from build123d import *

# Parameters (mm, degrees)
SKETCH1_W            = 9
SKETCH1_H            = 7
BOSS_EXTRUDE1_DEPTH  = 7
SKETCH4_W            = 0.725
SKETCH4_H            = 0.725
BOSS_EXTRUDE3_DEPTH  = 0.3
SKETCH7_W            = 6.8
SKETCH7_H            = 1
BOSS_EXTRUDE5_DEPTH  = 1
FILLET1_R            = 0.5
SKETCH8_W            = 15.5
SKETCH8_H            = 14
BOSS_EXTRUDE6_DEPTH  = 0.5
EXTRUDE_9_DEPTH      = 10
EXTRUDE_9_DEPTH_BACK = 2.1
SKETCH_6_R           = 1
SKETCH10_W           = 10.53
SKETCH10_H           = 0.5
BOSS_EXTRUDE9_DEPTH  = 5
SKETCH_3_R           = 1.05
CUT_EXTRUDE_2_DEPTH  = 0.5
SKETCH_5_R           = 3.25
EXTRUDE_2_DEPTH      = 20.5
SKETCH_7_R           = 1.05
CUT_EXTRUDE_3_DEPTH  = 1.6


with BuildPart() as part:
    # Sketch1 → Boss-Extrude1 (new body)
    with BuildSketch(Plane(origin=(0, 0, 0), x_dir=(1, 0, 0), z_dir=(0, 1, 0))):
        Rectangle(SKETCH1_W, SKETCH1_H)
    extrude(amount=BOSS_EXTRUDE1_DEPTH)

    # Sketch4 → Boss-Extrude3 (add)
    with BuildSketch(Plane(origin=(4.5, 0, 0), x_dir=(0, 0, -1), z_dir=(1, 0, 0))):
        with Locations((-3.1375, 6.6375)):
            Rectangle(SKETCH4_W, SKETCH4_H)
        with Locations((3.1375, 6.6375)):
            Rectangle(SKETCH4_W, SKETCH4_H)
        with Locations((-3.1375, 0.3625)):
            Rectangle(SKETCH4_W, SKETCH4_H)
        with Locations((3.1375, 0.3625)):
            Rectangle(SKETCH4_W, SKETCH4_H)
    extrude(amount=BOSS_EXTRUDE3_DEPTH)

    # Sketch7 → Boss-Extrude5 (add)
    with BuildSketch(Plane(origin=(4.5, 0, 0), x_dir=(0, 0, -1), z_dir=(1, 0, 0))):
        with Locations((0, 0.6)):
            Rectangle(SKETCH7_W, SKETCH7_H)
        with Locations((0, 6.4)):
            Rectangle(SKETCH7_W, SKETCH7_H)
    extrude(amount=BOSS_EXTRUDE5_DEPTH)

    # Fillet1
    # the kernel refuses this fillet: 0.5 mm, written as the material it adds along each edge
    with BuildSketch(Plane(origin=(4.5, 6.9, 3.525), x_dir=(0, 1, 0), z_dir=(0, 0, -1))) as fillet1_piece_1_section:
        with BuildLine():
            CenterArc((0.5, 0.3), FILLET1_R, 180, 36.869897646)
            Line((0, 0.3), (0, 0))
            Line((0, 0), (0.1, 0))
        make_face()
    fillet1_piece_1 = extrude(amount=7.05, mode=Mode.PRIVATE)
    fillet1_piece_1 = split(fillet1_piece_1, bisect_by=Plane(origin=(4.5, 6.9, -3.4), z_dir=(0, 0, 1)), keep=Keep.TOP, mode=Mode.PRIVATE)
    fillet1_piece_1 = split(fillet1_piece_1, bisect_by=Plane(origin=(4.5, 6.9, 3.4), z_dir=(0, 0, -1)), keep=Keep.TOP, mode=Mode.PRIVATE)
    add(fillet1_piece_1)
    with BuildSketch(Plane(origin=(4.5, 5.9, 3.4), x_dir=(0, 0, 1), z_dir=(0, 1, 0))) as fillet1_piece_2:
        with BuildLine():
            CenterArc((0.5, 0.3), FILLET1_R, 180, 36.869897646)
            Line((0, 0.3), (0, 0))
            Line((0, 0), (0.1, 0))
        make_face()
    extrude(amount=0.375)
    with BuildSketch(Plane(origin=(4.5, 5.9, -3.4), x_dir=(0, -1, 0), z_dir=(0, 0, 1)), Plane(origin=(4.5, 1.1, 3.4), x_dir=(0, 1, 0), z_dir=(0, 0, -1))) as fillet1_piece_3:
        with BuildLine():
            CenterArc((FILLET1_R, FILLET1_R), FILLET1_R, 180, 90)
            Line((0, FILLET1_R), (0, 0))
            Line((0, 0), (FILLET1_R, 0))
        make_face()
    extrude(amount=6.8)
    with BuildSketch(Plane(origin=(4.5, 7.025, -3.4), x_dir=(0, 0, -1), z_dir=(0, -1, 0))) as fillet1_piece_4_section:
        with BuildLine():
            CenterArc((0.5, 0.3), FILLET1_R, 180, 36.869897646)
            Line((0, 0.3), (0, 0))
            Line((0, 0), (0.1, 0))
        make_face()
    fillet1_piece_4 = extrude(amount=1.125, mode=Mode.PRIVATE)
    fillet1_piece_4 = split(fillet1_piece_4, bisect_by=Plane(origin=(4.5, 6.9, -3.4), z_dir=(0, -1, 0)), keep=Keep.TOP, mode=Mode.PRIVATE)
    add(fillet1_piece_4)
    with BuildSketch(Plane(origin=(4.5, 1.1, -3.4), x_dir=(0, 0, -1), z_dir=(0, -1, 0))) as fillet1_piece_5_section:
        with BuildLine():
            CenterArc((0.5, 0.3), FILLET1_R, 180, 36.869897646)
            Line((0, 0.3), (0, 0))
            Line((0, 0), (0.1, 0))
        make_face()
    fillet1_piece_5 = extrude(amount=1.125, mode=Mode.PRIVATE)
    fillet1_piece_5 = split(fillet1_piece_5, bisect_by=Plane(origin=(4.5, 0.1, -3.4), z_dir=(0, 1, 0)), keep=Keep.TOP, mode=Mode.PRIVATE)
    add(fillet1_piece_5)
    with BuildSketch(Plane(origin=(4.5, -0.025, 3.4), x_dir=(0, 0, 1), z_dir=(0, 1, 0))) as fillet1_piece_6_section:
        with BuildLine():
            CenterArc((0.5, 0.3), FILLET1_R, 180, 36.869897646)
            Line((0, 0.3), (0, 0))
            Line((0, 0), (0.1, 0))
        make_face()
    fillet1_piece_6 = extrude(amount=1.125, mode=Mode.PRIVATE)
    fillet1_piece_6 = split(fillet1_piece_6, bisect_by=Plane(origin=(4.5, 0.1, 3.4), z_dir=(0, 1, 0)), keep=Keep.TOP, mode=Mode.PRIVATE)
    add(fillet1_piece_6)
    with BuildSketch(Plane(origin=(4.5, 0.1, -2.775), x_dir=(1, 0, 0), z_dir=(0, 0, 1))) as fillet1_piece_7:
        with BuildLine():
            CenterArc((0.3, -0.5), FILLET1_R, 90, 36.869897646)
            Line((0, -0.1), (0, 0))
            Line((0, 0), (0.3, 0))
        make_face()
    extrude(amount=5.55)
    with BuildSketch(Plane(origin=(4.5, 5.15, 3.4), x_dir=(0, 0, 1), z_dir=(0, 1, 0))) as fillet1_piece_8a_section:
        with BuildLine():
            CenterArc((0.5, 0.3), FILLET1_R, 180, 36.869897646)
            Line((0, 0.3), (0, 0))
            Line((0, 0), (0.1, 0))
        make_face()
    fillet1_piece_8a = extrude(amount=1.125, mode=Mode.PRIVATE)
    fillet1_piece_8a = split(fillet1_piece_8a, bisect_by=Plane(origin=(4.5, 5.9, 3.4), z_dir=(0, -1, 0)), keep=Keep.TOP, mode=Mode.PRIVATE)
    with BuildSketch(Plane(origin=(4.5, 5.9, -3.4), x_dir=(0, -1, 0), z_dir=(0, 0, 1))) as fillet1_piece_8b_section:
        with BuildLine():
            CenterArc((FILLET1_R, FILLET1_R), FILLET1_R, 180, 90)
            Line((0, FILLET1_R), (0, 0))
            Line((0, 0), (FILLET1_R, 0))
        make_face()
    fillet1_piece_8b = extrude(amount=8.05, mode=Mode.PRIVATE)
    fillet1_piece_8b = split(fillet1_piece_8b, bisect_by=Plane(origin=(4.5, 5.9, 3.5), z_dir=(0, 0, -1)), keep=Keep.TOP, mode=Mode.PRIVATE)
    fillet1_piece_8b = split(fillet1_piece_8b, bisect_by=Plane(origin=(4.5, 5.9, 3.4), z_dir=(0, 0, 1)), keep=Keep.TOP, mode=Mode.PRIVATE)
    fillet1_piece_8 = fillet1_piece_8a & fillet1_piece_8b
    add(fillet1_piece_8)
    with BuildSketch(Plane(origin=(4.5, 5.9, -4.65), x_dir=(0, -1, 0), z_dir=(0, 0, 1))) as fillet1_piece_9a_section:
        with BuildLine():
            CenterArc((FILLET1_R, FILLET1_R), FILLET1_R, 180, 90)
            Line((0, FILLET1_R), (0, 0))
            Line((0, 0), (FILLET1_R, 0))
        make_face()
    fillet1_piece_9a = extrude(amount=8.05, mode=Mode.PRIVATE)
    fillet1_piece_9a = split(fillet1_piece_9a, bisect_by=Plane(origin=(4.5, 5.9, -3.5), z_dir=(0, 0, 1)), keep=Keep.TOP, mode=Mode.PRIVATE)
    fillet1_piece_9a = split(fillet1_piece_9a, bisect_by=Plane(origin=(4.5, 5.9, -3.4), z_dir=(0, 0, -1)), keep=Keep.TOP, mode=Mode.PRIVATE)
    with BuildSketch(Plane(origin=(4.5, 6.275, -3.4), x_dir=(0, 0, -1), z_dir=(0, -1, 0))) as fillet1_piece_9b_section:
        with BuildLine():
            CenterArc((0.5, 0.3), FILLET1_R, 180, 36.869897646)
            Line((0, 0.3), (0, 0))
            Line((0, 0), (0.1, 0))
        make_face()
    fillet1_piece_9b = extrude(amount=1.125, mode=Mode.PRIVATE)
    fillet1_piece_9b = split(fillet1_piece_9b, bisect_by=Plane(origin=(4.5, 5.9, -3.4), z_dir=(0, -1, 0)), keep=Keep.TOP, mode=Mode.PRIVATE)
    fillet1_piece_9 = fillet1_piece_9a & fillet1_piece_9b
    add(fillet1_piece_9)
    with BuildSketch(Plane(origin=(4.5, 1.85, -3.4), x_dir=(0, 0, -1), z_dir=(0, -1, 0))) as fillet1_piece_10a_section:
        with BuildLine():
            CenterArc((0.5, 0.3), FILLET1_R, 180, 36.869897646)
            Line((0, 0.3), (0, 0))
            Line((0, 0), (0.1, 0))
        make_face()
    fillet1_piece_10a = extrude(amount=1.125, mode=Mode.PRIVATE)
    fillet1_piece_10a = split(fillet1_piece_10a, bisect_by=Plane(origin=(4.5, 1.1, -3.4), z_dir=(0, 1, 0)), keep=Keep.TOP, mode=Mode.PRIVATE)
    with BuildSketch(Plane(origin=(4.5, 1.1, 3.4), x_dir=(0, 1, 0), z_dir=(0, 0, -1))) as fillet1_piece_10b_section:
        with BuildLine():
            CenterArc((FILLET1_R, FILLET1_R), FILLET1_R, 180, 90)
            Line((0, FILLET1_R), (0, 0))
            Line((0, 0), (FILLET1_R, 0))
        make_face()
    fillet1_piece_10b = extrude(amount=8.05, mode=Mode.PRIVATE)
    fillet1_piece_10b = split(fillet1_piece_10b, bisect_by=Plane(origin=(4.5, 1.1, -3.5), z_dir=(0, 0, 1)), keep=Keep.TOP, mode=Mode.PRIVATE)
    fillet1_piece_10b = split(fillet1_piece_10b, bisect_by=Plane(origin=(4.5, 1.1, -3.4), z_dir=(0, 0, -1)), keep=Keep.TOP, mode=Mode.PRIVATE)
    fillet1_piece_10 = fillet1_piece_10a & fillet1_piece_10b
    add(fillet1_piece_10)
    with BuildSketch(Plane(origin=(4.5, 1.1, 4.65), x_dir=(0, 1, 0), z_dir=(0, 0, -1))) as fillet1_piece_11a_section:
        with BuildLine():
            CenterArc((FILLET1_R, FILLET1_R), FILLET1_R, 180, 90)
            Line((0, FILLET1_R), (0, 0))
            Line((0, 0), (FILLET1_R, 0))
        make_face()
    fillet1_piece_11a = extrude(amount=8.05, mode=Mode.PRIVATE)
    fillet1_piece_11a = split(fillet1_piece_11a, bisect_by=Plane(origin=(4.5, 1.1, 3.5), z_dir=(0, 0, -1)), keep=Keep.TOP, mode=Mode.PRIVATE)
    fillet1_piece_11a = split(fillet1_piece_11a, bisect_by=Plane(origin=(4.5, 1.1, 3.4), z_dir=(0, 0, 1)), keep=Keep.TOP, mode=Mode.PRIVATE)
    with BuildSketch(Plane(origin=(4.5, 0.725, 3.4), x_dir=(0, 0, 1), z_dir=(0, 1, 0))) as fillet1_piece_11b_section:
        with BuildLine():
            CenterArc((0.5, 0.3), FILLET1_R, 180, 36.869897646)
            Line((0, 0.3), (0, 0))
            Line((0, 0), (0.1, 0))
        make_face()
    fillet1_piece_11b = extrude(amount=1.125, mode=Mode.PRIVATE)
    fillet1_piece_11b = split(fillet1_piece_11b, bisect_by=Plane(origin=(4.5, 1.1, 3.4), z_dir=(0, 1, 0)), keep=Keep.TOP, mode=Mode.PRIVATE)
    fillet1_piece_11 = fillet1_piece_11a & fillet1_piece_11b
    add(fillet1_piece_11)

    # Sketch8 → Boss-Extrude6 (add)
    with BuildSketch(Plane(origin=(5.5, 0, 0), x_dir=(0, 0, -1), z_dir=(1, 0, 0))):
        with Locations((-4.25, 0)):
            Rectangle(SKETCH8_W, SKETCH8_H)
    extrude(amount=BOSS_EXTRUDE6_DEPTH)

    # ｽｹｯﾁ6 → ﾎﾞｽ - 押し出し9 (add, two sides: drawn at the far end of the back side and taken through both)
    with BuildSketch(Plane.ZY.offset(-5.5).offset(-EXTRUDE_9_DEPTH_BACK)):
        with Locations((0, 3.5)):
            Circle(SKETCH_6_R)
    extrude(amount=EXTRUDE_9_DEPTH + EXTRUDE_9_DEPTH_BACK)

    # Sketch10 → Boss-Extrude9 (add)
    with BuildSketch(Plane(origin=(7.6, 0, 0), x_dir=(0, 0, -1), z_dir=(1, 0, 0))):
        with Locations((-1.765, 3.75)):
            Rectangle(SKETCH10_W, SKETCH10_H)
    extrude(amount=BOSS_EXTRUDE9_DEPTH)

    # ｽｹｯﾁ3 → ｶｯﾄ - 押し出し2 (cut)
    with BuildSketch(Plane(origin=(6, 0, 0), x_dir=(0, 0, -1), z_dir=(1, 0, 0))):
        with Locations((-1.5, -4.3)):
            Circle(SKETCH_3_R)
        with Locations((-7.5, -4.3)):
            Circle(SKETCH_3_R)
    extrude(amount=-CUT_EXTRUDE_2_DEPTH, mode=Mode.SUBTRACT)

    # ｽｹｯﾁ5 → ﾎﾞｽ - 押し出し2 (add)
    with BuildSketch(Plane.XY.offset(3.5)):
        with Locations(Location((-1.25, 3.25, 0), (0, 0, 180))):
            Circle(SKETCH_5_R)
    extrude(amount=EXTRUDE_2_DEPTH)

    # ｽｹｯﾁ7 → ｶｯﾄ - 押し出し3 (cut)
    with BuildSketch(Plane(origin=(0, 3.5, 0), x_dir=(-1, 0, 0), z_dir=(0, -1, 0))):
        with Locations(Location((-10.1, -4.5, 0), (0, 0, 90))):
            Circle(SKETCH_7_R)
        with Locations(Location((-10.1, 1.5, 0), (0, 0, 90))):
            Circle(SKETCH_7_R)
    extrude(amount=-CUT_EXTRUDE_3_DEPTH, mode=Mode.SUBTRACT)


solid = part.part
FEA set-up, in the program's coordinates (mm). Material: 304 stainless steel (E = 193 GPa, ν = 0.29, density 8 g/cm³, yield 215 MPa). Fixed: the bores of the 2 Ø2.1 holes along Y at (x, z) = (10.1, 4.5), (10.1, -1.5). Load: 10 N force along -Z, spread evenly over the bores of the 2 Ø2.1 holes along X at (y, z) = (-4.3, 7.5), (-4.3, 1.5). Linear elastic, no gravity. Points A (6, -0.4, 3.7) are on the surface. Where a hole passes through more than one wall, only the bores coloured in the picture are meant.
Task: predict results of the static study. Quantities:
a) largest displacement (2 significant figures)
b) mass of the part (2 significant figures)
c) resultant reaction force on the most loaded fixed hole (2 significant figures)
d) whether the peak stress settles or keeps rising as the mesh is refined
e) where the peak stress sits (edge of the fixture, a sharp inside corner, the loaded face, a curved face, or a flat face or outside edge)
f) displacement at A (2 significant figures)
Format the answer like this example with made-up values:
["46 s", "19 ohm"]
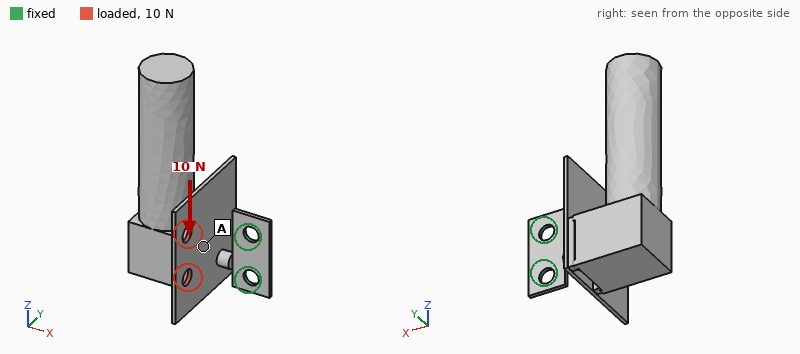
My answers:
["0.24 mm", "10 g", "16 N", "keeps rising", "a sharp inside corner", "0.055 mm"]
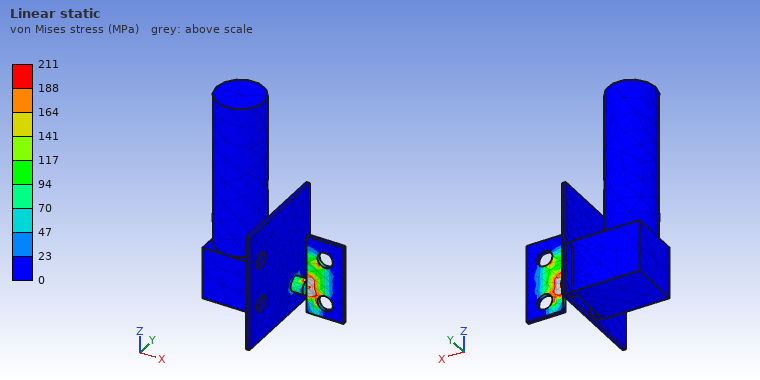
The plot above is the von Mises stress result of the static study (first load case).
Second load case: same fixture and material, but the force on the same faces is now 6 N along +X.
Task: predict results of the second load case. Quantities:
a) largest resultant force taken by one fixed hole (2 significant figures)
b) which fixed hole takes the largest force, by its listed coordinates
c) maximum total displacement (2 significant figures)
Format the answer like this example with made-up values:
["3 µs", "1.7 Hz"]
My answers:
["6.2 N", "(10.1, 4.5)", "0.20 mm"]
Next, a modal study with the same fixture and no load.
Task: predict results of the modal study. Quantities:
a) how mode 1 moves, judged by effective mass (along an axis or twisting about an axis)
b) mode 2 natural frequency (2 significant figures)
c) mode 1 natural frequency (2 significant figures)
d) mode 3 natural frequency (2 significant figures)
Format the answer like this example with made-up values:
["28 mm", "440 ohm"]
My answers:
["along Y", "640 Hz", "260 Hz", "700 Hz"]
